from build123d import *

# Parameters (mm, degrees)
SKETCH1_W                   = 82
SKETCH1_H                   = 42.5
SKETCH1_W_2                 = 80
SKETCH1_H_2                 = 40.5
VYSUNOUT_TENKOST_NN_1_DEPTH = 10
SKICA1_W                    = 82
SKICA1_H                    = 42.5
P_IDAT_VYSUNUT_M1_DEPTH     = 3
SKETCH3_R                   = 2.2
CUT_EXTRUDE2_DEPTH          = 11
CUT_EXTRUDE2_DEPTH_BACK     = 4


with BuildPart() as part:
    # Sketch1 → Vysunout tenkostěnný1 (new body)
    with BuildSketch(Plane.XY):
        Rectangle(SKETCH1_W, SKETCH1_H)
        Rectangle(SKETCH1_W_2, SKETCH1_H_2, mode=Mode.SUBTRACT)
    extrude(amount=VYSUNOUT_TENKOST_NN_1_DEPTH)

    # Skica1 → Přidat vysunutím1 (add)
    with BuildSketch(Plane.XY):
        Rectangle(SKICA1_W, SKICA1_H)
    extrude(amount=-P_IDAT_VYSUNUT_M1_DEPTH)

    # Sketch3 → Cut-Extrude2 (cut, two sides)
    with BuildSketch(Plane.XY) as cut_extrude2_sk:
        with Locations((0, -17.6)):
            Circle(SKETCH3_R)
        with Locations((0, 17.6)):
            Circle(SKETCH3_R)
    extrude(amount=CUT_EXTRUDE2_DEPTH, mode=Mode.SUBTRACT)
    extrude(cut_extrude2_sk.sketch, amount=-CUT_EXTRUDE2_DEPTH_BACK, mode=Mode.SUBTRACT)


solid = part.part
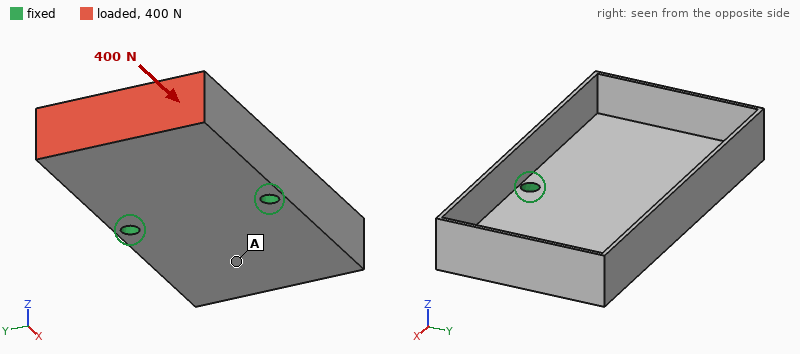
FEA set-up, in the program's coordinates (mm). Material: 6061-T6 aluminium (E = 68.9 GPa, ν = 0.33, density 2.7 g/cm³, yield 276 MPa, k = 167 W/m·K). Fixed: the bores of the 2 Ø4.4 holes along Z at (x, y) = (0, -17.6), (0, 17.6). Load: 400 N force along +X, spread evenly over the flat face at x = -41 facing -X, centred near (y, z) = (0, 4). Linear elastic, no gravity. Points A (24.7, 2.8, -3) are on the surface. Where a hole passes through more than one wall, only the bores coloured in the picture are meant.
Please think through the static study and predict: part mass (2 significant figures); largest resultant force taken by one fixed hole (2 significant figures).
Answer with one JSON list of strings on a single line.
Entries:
["35 g", "200 N"]
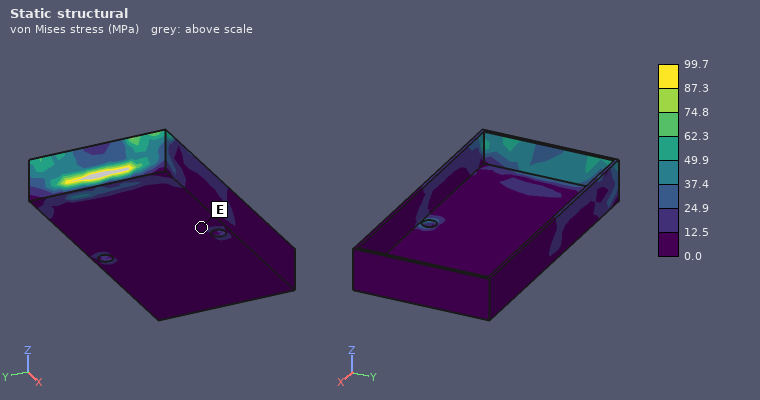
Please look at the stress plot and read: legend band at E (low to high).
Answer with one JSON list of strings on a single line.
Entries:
["0.0 to 12.5 MPa"]
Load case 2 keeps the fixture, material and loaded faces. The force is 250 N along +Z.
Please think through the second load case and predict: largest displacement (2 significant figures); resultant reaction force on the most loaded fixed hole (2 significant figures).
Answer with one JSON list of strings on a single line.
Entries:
["0.24 mm", "130 N"]
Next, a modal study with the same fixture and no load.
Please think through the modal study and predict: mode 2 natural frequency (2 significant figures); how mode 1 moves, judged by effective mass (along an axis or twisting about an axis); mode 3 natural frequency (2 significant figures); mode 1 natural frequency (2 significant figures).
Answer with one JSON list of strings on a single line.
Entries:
["3200 Hz", "twisting about Y", "3300 Hz", "1800 Hz"]
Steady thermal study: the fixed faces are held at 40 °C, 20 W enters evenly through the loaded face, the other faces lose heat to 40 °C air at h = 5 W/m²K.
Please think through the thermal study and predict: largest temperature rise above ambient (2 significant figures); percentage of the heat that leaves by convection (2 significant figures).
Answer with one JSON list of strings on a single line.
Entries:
["46 K", "3.4 %"]
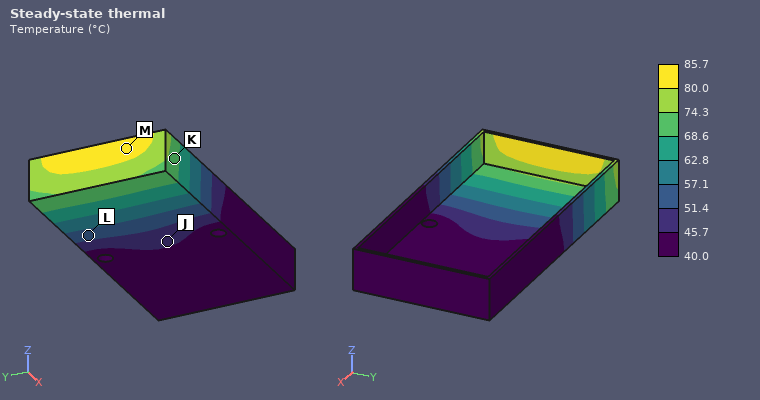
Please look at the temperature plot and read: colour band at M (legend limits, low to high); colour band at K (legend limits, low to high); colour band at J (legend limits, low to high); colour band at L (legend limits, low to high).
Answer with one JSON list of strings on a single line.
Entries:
["80.0 to 85.7 °C", "68.6 to 74.3 °C", "45.7 to 51.4 °C", "51.4 to 57.1 °C"]
